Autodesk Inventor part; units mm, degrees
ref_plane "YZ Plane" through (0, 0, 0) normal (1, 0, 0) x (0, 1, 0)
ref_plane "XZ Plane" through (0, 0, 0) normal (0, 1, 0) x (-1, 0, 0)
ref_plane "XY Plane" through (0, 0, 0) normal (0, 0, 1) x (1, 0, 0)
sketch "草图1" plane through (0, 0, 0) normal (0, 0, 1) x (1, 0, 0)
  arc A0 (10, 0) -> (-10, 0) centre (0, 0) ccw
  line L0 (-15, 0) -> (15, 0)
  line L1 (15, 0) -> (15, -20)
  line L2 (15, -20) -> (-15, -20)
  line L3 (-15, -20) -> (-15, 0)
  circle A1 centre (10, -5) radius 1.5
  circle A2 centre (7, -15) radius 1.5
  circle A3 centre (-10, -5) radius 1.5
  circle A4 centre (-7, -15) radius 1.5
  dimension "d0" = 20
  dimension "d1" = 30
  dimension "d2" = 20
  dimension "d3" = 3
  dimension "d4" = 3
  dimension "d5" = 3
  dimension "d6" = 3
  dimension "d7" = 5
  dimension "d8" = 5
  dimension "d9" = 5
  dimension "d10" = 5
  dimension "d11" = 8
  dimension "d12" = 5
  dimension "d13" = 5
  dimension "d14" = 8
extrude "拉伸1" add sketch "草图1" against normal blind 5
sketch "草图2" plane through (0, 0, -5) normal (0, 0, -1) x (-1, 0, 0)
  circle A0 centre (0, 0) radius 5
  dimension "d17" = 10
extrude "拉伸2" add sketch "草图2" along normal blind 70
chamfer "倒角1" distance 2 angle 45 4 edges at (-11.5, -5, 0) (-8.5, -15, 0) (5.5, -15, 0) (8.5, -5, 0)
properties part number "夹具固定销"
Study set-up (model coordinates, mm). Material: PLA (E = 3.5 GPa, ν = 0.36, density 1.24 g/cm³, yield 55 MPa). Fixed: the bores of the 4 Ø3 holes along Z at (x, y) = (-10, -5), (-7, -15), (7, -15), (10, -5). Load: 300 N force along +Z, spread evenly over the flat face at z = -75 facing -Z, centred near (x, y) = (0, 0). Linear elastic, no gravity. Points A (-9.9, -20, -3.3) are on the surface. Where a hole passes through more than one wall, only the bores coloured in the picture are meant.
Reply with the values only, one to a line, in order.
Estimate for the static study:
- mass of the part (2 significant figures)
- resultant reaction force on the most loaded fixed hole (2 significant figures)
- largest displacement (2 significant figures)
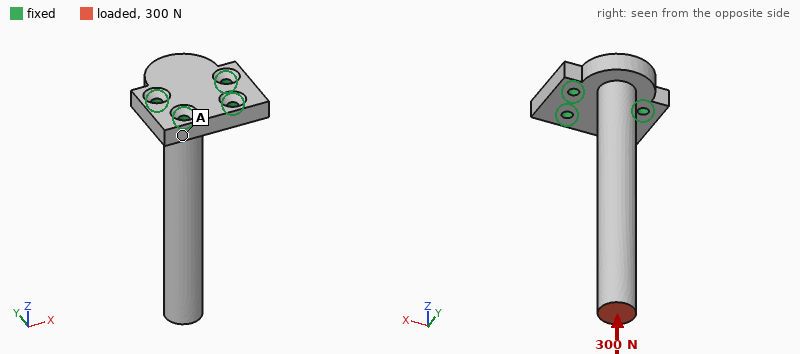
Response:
11 g
180 N
0.77 mm
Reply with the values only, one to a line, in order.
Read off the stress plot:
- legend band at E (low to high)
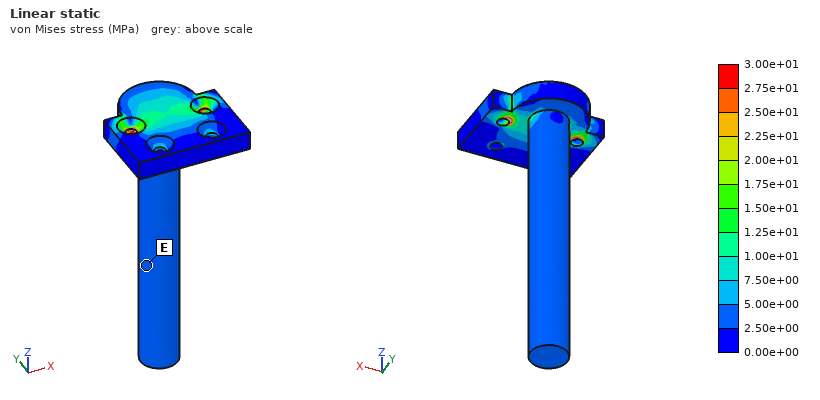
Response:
2.50e+00 to 5.00e+00 MPa
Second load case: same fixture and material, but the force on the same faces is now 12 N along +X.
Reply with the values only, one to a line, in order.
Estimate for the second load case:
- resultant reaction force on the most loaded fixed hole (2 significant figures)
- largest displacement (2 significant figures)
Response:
49 N
1.00 mm
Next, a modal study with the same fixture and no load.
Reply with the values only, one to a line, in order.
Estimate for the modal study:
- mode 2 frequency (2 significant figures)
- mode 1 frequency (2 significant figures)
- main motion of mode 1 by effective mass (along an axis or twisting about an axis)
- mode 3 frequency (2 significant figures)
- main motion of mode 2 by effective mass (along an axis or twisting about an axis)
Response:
410 Hz
350 Hz
along Y
2200 Hz
along X
